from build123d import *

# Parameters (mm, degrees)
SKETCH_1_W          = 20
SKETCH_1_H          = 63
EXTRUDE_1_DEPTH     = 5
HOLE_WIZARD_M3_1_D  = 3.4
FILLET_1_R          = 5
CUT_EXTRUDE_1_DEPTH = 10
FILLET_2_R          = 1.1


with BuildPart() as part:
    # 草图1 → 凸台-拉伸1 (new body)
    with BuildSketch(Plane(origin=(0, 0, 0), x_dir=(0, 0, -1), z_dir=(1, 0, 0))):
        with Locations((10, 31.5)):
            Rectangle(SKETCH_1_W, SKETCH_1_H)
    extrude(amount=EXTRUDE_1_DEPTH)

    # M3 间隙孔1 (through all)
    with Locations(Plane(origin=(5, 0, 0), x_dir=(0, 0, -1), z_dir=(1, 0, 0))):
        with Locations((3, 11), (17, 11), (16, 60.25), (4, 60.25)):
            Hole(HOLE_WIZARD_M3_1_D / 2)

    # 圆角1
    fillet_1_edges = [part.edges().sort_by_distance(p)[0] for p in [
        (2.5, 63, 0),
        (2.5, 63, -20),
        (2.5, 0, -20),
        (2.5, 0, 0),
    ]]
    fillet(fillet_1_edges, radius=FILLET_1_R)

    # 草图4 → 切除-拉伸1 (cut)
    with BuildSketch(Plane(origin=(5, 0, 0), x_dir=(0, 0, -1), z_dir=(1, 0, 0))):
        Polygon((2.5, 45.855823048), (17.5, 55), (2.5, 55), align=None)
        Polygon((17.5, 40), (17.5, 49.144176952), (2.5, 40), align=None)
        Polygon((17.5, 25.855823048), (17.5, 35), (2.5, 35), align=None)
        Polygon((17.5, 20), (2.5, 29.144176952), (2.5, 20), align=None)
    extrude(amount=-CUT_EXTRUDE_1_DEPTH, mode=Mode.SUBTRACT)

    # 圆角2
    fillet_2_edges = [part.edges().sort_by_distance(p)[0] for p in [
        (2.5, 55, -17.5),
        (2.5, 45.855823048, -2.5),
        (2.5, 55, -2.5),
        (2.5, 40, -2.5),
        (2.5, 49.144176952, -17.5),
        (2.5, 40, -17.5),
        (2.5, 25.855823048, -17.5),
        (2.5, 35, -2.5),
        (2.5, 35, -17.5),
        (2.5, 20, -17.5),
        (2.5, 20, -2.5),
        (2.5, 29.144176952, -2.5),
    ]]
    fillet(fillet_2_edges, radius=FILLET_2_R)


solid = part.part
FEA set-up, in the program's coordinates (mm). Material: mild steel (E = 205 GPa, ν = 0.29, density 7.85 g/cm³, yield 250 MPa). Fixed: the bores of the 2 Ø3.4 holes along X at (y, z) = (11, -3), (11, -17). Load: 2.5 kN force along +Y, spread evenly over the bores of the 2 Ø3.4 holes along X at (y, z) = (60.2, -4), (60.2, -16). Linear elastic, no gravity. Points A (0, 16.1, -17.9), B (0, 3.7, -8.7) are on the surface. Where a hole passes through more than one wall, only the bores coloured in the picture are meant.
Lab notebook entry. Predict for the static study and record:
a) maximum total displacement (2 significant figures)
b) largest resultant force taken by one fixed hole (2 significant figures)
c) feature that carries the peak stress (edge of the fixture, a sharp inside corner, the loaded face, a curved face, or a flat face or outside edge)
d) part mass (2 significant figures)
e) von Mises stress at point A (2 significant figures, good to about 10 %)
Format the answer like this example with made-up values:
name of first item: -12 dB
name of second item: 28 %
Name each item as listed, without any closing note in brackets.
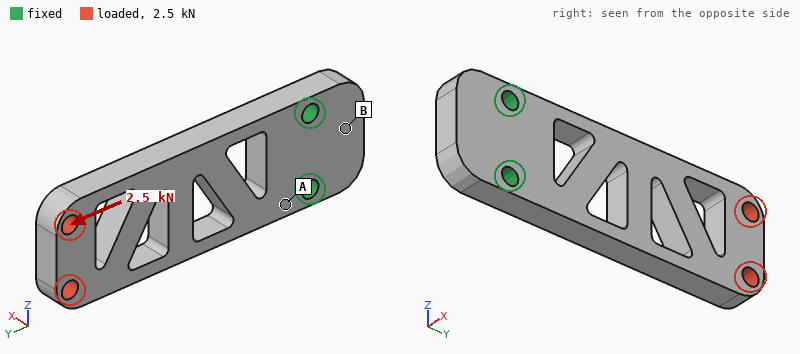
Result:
maximum total displacement: 19 µm
largest resultant force taken by one fixed hole: 1.3 kN
feature that carries the peak stress: a curved face
part mass: 37 g
von Mises stress at point A: 47 MPa
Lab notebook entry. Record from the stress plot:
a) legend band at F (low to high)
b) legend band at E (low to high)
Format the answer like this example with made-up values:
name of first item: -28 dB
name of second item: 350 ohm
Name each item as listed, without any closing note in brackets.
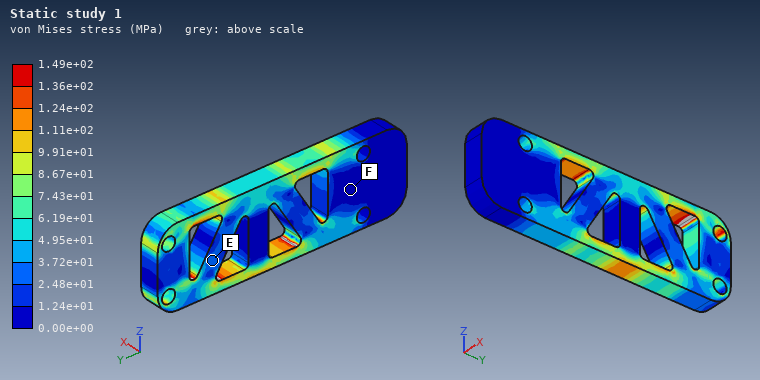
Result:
legend band at F: 0.00e+00 to 1.24e+01 MPa
legend band at E: 2.48e+01 to 3.72e+01 MPa
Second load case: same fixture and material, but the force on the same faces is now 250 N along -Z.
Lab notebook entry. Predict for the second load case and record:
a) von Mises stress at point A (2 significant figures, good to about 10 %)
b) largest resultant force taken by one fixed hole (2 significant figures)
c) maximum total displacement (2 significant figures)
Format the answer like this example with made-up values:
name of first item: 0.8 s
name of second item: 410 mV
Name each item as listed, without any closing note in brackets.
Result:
von Mises stress at point A: 31 MPa
largest resultant force taken by one fixed hole: 810 N
maximum total displacement: 30 µm
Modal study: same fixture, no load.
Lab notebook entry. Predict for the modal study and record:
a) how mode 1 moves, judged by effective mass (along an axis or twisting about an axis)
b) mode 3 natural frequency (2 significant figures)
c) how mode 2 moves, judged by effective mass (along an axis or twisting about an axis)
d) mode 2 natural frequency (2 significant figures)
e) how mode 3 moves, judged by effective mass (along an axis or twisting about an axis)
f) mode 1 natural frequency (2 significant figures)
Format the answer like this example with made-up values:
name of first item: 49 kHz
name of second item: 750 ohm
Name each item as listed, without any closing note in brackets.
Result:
how mode 1 moves, judged by effective mass: along X
mode 3 natural frequency: 6000 Hz
how mode 2 moves, judged by effective mass: along Z
mode 2 natural frequency: 5000 Hz
how mode 3 moves, judged by effective mass: twisting about Y
mode 1 natural frequency: 1300 Hz
